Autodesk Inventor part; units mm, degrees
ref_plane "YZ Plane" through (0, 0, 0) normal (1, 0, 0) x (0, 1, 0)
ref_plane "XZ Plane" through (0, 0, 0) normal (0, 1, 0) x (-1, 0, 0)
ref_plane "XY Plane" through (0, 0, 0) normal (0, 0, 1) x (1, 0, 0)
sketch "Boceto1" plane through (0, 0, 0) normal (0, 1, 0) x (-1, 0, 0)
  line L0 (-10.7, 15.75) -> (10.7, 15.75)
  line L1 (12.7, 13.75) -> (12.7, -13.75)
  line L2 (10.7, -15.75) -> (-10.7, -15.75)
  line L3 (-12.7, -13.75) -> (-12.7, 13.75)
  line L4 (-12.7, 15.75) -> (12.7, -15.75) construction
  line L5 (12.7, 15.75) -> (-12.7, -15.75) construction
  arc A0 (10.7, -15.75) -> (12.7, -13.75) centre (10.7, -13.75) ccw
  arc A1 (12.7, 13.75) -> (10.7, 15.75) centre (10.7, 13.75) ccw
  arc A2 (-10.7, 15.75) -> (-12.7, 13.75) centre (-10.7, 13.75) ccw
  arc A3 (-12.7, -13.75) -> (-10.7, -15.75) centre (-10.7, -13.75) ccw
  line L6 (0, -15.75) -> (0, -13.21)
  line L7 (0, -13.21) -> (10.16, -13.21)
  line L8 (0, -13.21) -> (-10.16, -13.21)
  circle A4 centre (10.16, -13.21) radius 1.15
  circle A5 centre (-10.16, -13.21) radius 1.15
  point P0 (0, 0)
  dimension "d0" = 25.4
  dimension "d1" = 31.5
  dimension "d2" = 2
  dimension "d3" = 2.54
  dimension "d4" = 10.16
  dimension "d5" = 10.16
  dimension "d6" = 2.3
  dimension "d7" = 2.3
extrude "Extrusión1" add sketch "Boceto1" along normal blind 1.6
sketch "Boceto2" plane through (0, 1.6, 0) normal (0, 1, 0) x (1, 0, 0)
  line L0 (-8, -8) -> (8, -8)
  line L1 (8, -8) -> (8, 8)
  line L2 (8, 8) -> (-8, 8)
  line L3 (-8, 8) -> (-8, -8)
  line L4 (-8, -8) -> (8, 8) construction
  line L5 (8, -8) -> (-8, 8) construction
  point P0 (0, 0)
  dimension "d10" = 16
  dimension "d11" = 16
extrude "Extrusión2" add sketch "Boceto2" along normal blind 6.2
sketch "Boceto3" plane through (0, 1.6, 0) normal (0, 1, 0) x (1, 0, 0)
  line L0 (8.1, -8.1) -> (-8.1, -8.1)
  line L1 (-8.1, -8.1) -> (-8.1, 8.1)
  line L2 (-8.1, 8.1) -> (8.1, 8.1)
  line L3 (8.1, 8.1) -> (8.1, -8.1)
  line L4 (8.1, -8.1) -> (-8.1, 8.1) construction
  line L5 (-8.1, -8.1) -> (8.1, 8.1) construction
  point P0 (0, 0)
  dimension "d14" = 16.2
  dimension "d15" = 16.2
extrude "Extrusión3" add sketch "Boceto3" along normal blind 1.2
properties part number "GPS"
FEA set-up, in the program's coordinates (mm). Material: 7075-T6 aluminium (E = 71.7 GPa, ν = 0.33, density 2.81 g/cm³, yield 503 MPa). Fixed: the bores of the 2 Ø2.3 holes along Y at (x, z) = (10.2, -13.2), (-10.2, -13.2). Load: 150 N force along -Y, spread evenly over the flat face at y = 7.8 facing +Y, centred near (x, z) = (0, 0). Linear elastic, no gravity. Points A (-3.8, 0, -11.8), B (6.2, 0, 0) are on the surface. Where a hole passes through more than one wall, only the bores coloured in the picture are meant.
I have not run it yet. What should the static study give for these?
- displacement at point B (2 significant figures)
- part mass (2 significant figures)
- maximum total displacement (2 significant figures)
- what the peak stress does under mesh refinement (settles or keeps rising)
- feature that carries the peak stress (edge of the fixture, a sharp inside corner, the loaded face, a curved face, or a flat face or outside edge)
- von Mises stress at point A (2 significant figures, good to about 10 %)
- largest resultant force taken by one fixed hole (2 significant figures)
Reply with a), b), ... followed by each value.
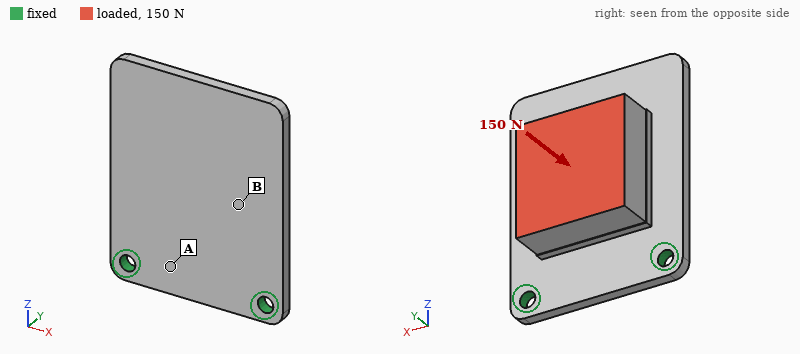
a) 0.18 mm
b) 8.0 g
c) 0.45 mm
d) keeps rising
e) edge of the fixture
f) 73 MPa
g) 75 N
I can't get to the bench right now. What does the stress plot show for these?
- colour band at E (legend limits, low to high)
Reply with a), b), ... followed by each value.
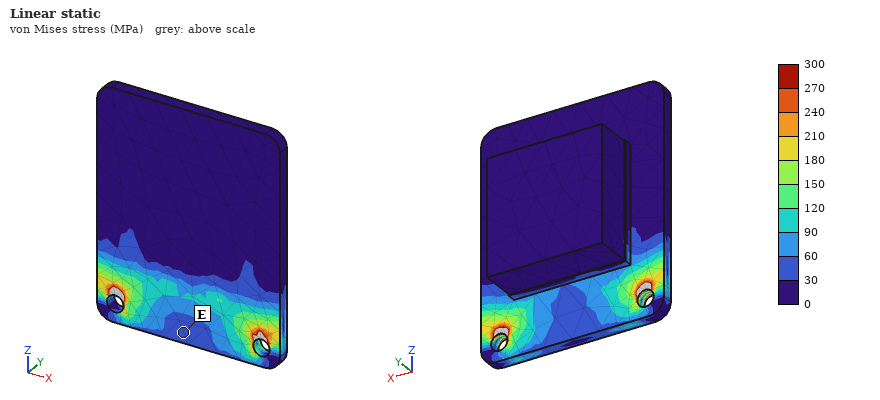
a) 30 to 60 MPa
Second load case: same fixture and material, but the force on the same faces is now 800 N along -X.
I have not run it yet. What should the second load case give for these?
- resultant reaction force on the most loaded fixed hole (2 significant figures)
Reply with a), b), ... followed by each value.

a) 710 N
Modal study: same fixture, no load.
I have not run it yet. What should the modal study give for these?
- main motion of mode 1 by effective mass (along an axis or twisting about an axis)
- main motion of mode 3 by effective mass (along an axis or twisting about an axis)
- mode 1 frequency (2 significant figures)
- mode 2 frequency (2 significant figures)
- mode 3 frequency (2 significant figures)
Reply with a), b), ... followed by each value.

a) along Y
b) along Y
c) 1300 Hz
d) 8500 Hz
e) 13 kHz
